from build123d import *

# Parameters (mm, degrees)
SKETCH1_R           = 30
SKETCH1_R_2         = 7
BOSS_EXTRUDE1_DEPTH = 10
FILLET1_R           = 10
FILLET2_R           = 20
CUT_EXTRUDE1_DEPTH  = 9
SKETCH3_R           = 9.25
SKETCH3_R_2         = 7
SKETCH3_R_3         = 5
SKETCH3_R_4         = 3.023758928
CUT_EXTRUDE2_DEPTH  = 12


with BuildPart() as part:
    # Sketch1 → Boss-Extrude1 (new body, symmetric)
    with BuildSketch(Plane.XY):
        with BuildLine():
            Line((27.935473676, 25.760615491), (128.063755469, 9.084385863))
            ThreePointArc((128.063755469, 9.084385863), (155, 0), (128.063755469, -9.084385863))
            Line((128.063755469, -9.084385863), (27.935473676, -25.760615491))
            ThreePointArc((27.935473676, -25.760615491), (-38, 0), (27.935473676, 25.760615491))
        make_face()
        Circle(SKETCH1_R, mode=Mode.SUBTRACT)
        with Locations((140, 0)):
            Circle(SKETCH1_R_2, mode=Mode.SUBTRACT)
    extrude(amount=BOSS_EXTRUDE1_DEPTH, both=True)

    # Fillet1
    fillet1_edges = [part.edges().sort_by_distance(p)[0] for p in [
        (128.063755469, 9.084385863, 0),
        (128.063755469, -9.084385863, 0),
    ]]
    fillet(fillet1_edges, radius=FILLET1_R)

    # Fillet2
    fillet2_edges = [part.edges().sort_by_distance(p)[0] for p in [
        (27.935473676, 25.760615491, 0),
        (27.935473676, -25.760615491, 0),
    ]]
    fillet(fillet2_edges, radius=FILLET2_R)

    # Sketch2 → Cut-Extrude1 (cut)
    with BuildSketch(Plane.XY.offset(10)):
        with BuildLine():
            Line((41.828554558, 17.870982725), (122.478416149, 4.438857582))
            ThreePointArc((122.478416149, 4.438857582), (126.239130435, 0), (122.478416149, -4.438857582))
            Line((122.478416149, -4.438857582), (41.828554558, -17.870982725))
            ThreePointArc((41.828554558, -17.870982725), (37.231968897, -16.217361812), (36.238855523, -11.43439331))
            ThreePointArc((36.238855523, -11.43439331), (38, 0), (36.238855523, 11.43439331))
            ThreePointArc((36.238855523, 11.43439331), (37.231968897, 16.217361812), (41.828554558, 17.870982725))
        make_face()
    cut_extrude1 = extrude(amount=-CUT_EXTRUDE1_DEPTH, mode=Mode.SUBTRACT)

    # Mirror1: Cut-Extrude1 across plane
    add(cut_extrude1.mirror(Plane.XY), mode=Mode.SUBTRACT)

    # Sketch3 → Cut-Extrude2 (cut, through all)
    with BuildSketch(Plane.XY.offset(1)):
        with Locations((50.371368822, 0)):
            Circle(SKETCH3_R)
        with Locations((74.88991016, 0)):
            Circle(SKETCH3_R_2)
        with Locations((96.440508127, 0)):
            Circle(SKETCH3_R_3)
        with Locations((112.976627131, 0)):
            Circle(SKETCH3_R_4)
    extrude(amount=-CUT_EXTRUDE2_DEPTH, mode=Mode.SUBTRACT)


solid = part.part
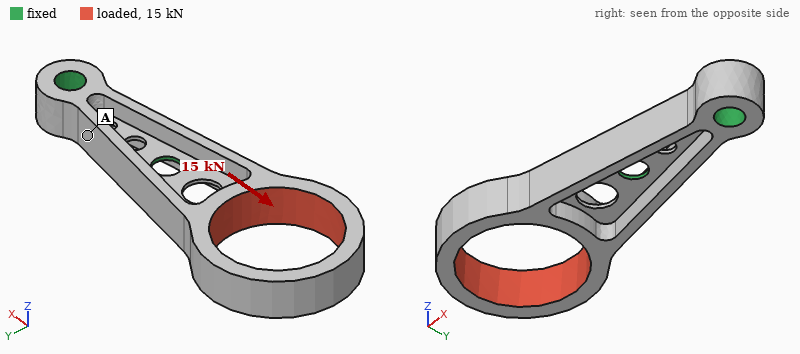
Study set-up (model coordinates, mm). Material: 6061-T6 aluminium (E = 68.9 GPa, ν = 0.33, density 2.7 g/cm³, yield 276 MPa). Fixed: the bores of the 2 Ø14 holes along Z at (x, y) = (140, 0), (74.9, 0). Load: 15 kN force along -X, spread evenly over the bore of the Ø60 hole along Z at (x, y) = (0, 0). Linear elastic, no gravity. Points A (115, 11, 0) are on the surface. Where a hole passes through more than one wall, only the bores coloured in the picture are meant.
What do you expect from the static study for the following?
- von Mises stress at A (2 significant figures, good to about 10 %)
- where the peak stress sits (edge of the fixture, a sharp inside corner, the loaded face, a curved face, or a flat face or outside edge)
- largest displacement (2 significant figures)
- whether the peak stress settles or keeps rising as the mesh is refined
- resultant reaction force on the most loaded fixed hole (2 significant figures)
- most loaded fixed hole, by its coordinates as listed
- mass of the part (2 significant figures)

21 MPa
edge of the fixture
0.30 mm
keeps rising
9.1 kN
(74.9, 0)
190 g
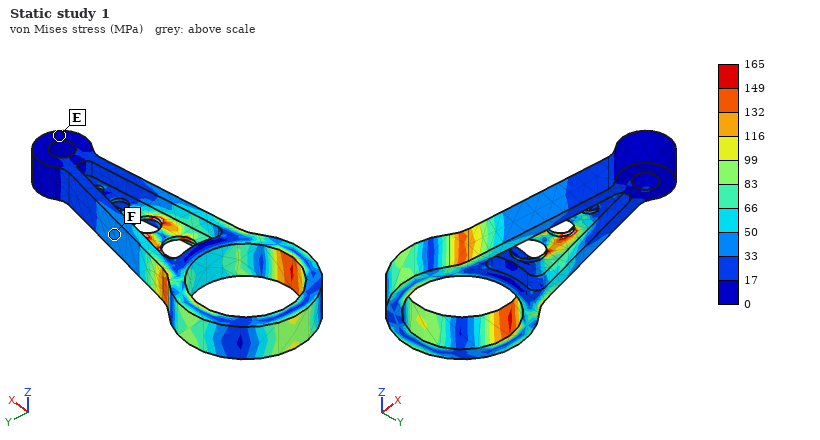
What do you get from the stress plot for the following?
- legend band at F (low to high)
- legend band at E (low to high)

33 to 50 MPa
0 to 17 MPa
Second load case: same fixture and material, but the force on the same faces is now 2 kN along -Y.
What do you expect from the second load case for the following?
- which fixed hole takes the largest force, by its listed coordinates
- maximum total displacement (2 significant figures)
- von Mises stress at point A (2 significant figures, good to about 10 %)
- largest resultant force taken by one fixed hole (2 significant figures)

(74.9, 0)
0.60 mm
20 MPa
3.5 kN
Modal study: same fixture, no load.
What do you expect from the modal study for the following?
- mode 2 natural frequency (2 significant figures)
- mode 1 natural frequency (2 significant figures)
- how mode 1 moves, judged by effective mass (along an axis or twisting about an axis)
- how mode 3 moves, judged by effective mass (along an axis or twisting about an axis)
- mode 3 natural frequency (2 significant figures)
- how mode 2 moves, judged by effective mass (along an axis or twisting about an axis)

940 Hz
600 Hz
along Z
along Y
1100 Hz
twisting about X
